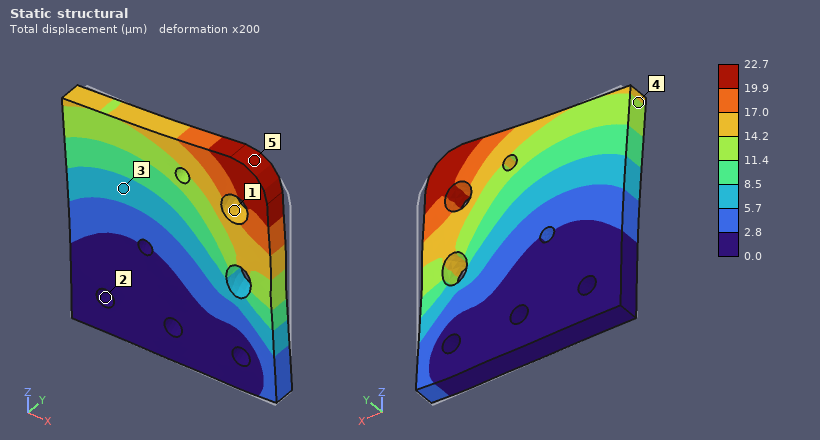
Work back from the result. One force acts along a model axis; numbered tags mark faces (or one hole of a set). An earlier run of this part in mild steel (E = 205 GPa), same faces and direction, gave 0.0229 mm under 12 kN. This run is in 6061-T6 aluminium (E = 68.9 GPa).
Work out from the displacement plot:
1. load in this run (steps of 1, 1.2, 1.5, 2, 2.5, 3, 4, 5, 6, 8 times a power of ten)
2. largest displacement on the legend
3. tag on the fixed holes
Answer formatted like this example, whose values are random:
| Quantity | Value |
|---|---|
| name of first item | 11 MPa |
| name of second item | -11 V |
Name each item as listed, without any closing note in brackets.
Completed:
| Quantity | Value |
|---|---|
| load in this run | 4 kN |
| largest displacement on the legend | 22.7 µm |
| tag on the fixed holes | 2 |
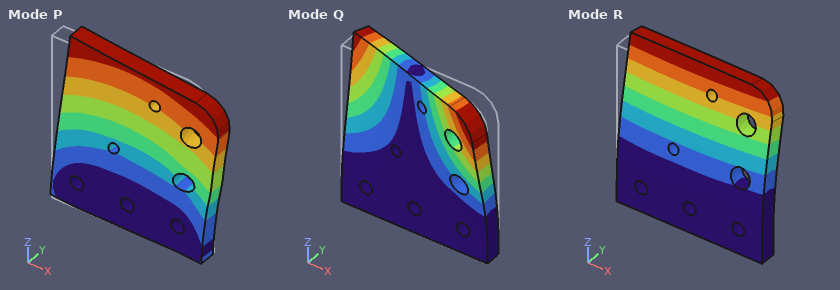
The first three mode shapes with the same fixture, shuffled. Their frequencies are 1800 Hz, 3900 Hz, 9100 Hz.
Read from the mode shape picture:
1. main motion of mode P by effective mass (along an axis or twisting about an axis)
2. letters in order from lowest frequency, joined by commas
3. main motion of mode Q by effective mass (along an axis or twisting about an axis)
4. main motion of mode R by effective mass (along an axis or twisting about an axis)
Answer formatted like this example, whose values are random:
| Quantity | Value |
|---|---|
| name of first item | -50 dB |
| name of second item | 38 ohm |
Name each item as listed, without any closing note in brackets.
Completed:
| Quantity | Value |
|---|---|
| main motion of mode P by effective mass | along X |
| letters in order from lowest frequency, joined by commas | R, Q, P |
| main motion of mode Q by effective mass | twisting about Z |
| main motion of mode R by effective mass | along Y |
